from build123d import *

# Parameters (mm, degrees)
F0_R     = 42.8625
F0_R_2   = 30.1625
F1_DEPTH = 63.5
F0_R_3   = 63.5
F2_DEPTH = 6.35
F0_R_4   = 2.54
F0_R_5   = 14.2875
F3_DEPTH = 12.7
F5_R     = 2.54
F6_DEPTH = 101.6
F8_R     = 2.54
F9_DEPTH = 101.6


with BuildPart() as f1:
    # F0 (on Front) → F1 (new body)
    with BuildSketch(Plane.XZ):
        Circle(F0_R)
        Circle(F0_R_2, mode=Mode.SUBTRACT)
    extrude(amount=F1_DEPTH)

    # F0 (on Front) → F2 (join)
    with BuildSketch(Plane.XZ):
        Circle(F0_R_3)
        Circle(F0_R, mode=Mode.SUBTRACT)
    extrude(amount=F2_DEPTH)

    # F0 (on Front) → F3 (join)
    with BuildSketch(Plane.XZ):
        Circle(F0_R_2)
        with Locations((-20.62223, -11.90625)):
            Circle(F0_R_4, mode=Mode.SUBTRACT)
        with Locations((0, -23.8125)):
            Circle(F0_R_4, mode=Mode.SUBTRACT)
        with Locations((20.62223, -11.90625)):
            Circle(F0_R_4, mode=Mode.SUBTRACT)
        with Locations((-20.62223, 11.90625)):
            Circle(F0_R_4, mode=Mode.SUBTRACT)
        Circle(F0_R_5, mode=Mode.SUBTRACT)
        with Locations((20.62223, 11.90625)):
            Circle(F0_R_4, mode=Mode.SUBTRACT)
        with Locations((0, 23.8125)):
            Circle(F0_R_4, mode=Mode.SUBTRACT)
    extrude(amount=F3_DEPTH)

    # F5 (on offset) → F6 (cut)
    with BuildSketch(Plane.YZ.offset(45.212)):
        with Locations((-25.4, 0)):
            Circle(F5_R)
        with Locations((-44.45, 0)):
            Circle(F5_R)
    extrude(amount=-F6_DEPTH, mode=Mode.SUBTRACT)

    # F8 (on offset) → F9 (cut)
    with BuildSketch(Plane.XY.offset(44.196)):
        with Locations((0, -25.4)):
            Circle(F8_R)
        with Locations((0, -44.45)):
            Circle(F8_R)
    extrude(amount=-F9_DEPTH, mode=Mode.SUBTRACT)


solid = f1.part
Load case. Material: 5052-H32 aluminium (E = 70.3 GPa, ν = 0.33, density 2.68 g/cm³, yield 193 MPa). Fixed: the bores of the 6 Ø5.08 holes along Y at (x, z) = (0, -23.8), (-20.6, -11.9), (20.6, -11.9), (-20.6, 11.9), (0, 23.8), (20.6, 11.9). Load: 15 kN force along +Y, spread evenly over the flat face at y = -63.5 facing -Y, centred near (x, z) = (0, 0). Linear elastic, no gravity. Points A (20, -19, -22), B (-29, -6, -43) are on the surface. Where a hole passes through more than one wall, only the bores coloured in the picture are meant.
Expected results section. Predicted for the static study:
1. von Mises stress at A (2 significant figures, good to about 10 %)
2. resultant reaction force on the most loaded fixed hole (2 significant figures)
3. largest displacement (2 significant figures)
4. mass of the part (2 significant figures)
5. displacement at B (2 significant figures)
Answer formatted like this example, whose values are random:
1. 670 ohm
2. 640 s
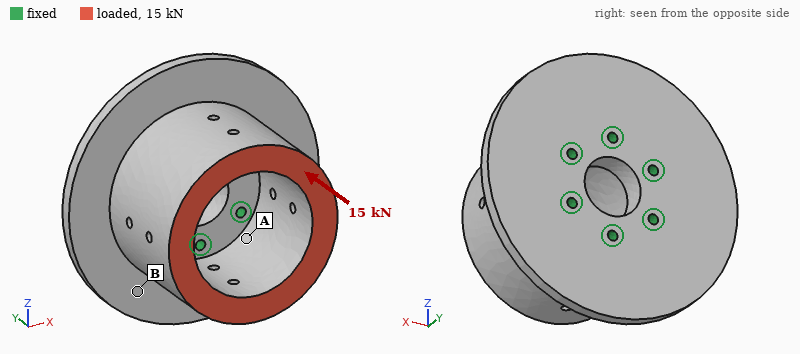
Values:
1. 13 MPa
2. 2.5 kN
3. 12 µm
4. 680 g
5. 9.2 µm
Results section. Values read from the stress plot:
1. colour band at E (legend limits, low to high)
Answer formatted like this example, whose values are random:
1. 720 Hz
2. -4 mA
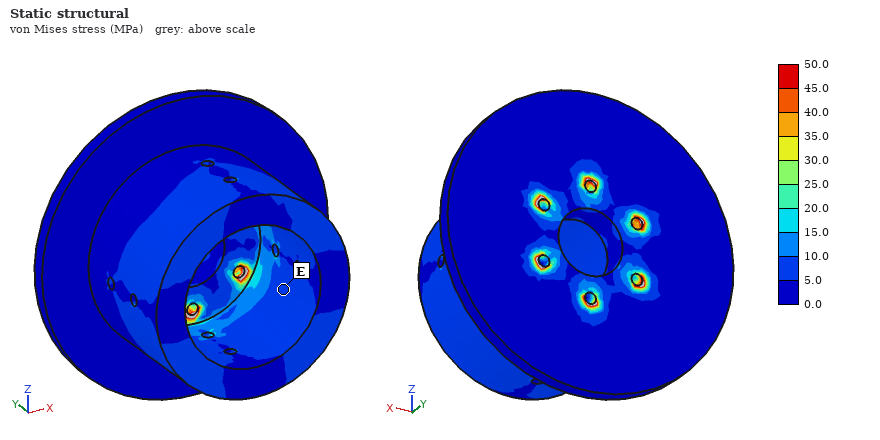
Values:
1. 5.0 to 10.0 MPa
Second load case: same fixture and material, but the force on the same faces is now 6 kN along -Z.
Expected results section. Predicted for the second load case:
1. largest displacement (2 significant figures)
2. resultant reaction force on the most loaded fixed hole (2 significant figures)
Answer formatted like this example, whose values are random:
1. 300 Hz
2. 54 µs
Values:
1. 38 µm
2. 3.4 kN
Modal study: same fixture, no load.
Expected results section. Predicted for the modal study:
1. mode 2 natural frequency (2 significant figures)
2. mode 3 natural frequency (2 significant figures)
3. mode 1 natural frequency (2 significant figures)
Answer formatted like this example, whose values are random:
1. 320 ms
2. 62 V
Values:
1. 4500 Hz
2. 6500 Hz
3. 4500 Hz
